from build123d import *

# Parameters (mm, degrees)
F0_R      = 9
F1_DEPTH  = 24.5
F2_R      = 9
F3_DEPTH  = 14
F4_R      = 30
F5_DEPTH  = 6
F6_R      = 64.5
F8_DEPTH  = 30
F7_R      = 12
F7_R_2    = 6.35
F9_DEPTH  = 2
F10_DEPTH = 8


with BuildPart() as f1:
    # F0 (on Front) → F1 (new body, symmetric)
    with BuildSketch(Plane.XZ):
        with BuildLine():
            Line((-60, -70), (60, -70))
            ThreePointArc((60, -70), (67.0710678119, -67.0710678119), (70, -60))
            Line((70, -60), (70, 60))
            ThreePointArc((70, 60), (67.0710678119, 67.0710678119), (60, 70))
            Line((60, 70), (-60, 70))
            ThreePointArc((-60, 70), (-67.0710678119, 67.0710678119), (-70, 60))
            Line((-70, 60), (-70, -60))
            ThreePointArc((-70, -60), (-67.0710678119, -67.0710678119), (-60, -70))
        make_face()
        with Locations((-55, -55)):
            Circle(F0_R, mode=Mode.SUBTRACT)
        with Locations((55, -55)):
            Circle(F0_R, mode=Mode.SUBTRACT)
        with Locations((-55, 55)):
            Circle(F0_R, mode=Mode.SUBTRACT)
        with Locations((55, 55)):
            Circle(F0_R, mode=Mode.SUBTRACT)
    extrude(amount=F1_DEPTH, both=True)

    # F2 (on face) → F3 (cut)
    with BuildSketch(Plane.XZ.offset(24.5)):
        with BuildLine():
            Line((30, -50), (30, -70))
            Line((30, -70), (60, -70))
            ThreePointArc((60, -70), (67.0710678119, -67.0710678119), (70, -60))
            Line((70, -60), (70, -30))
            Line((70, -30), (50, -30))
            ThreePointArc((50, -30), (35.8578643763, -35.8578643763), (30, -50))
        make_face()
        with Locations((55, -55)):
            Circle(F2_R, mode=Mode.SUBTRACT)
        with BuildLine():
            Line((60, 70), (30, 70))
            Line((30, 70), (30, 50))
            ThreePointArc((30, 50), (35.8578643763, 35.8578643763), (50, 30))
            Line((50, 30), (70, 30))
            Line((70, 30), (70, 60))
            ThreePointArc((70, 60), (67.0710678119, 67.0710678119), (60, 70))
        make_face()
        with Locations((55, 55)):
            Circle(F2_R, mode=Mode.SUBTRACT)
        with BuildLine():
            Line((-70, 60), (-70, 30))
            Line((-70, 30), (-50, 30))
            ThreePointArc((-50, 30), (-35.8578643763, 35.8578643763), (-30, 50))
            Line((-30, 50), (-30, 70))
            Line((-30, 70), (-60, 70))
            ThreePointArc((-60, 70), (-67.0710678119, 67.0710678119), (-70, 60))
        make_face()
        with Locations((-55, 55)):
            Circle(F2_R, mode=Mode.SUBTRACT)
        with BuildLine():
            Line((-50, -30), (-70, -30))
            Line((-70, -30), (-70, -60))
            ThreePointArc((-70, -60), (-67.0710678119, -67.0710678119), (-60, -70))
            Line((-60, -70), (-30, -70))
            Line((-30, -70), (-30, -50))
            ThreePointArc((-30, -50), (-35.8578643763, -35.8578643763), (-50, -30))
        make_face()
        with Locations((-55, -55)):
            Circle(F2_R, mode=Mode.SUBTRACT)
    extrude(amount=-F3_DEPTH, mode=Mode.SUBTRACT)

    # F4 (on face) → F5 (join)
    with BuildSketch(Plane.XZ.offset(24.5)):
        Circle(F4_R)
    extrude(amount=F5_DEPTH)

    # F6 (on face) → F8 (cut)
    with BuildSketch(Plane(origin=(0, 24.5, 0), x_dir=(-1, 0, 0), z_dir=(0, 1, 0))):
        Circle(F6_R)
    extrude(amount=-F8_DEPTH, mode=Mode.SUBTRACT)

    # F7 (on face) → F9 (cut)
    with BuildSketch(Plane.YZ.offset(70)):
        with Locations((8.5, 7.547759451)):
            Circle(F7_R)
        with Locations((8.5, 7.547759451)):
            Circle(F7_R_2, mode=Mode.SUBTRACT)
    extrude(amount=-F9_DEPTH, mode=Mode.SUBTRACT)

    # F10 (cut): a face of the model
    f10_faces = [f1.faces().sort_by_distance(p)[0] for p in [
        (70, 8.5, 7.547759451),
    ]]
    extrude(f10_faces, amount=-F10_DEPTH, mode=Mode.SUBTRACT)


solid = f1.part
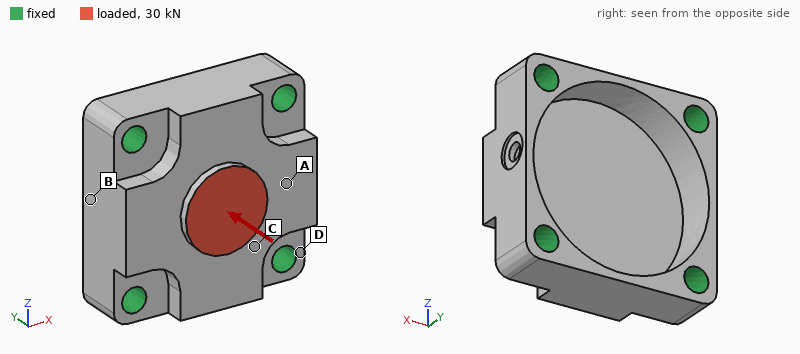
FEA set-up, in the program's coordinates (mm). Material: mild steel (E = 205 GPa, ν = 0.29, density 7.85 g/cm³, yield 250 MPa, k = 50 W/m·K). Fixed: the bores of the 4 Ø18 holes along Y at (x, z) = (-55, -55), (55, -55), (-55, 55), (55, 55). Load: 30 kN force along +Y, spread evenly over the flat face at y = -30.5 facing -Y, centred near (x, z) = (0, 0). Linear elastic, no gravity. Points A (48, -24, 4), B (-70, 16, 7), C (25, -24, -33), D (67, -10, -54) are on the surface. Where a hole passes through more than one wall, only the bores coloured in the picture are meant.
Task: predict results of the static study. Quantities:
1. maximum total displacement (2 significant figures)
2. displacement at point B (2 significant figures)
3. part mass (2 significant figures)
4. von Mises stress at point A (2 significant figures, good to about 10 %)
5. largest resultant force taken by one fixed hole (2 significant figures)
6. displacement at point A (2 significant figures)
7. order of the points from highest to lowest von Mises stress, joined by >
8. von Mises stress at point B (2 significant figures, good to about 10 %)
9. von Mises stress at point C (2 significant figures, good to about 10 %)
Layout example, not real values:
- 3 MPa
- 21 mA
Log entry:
- 26 µm
- 4.6 µm
- 3.6 kg
- 18 MPa
- 11 kN
- 13 µm
- C > A > B > D
- 12 MPa
- 25 MPa
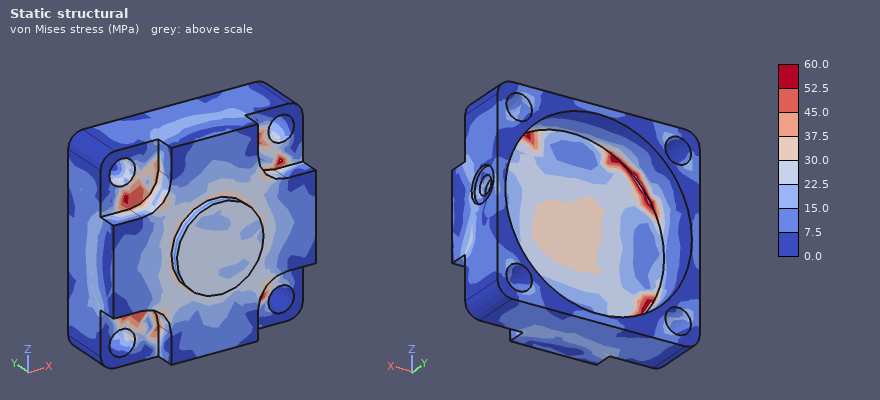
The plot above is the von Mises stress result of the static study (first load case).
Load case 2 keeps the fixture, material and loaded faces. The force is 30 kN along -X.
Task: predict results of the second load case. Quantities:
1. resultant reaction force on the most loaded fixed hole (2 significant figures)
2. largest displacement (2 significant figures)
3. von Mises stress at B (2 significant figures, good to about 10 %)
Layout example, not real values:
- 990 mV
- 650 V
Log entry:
- 9.0 kN
- 10 µm
- 7.4 MPa
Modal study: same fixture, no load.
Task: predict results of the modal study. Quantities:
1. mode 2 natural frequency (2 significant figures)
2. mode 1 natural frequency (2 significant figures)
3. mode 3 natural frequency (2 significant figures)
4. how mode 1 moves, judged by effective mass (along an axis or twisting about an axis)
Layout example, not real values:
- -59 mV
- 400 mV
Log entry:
- 9000 Hz
- 5500 Hz
- 9000 Hz
- along Y
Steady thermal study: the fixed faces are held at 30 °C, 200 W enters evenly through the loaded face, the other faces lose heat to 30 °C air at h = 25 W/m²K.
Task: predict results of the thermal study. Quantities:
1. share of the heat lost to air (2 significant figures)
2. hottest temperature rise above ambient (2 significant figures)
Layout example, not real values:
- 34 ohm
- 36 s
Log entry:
- 18 %
- 78 K
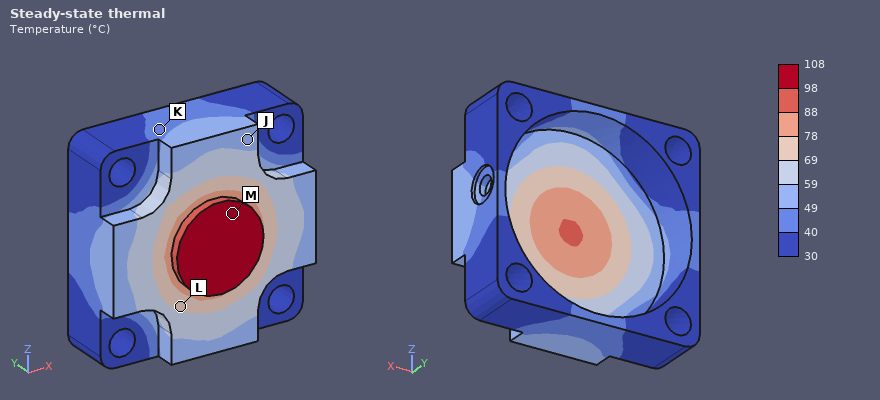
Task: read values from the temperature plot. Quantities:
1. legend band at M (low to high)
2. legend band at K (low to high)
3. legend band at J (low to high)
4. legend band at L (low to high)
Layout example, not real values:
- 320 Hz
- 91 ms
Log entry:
- 98 to 108 °C
- 40 to 49 °C
- 49 to 59 °C
- 69 to 78 °C
